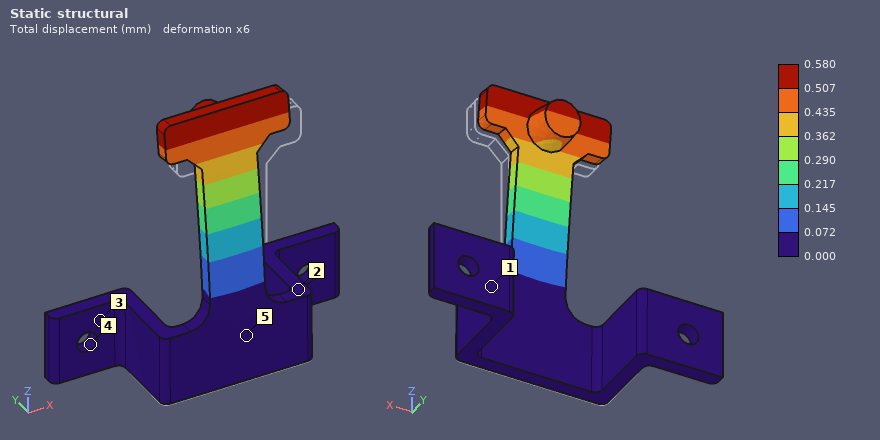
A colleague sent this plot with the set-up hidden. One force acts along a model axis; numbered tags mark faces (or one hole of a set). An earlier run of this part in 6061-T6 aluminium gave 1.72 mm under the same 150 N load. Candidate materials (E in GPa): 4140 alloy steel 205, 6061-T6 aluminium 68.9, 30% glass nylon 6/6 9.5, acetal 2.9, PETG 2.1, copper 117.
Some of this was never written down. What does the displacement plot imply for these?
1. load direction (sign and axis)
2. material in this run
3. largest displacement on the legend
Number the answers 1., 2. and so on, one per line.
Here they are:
1. +Y
2. 4140 alloy steel
3. 0.580 mm
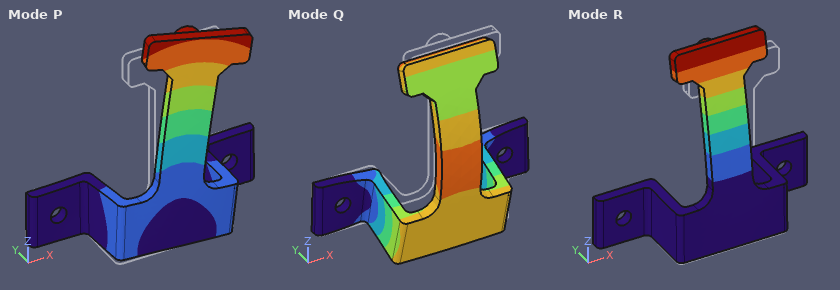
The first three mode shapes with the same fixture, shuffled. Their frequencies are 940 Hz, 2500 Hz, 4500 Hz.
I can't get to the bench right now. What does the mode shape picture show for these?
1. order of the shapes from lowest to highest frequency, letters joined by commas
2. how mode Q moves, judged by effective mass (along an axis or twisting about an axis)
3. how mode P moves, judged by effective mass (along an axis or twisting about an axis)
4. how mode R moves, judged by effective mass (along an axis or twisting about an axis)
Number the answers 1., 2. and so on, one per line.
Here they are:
1. R, P, Q
2. along Z
3. along X
4. along Y
